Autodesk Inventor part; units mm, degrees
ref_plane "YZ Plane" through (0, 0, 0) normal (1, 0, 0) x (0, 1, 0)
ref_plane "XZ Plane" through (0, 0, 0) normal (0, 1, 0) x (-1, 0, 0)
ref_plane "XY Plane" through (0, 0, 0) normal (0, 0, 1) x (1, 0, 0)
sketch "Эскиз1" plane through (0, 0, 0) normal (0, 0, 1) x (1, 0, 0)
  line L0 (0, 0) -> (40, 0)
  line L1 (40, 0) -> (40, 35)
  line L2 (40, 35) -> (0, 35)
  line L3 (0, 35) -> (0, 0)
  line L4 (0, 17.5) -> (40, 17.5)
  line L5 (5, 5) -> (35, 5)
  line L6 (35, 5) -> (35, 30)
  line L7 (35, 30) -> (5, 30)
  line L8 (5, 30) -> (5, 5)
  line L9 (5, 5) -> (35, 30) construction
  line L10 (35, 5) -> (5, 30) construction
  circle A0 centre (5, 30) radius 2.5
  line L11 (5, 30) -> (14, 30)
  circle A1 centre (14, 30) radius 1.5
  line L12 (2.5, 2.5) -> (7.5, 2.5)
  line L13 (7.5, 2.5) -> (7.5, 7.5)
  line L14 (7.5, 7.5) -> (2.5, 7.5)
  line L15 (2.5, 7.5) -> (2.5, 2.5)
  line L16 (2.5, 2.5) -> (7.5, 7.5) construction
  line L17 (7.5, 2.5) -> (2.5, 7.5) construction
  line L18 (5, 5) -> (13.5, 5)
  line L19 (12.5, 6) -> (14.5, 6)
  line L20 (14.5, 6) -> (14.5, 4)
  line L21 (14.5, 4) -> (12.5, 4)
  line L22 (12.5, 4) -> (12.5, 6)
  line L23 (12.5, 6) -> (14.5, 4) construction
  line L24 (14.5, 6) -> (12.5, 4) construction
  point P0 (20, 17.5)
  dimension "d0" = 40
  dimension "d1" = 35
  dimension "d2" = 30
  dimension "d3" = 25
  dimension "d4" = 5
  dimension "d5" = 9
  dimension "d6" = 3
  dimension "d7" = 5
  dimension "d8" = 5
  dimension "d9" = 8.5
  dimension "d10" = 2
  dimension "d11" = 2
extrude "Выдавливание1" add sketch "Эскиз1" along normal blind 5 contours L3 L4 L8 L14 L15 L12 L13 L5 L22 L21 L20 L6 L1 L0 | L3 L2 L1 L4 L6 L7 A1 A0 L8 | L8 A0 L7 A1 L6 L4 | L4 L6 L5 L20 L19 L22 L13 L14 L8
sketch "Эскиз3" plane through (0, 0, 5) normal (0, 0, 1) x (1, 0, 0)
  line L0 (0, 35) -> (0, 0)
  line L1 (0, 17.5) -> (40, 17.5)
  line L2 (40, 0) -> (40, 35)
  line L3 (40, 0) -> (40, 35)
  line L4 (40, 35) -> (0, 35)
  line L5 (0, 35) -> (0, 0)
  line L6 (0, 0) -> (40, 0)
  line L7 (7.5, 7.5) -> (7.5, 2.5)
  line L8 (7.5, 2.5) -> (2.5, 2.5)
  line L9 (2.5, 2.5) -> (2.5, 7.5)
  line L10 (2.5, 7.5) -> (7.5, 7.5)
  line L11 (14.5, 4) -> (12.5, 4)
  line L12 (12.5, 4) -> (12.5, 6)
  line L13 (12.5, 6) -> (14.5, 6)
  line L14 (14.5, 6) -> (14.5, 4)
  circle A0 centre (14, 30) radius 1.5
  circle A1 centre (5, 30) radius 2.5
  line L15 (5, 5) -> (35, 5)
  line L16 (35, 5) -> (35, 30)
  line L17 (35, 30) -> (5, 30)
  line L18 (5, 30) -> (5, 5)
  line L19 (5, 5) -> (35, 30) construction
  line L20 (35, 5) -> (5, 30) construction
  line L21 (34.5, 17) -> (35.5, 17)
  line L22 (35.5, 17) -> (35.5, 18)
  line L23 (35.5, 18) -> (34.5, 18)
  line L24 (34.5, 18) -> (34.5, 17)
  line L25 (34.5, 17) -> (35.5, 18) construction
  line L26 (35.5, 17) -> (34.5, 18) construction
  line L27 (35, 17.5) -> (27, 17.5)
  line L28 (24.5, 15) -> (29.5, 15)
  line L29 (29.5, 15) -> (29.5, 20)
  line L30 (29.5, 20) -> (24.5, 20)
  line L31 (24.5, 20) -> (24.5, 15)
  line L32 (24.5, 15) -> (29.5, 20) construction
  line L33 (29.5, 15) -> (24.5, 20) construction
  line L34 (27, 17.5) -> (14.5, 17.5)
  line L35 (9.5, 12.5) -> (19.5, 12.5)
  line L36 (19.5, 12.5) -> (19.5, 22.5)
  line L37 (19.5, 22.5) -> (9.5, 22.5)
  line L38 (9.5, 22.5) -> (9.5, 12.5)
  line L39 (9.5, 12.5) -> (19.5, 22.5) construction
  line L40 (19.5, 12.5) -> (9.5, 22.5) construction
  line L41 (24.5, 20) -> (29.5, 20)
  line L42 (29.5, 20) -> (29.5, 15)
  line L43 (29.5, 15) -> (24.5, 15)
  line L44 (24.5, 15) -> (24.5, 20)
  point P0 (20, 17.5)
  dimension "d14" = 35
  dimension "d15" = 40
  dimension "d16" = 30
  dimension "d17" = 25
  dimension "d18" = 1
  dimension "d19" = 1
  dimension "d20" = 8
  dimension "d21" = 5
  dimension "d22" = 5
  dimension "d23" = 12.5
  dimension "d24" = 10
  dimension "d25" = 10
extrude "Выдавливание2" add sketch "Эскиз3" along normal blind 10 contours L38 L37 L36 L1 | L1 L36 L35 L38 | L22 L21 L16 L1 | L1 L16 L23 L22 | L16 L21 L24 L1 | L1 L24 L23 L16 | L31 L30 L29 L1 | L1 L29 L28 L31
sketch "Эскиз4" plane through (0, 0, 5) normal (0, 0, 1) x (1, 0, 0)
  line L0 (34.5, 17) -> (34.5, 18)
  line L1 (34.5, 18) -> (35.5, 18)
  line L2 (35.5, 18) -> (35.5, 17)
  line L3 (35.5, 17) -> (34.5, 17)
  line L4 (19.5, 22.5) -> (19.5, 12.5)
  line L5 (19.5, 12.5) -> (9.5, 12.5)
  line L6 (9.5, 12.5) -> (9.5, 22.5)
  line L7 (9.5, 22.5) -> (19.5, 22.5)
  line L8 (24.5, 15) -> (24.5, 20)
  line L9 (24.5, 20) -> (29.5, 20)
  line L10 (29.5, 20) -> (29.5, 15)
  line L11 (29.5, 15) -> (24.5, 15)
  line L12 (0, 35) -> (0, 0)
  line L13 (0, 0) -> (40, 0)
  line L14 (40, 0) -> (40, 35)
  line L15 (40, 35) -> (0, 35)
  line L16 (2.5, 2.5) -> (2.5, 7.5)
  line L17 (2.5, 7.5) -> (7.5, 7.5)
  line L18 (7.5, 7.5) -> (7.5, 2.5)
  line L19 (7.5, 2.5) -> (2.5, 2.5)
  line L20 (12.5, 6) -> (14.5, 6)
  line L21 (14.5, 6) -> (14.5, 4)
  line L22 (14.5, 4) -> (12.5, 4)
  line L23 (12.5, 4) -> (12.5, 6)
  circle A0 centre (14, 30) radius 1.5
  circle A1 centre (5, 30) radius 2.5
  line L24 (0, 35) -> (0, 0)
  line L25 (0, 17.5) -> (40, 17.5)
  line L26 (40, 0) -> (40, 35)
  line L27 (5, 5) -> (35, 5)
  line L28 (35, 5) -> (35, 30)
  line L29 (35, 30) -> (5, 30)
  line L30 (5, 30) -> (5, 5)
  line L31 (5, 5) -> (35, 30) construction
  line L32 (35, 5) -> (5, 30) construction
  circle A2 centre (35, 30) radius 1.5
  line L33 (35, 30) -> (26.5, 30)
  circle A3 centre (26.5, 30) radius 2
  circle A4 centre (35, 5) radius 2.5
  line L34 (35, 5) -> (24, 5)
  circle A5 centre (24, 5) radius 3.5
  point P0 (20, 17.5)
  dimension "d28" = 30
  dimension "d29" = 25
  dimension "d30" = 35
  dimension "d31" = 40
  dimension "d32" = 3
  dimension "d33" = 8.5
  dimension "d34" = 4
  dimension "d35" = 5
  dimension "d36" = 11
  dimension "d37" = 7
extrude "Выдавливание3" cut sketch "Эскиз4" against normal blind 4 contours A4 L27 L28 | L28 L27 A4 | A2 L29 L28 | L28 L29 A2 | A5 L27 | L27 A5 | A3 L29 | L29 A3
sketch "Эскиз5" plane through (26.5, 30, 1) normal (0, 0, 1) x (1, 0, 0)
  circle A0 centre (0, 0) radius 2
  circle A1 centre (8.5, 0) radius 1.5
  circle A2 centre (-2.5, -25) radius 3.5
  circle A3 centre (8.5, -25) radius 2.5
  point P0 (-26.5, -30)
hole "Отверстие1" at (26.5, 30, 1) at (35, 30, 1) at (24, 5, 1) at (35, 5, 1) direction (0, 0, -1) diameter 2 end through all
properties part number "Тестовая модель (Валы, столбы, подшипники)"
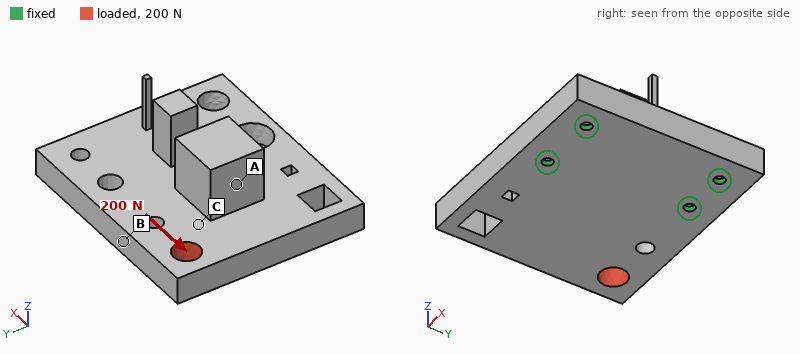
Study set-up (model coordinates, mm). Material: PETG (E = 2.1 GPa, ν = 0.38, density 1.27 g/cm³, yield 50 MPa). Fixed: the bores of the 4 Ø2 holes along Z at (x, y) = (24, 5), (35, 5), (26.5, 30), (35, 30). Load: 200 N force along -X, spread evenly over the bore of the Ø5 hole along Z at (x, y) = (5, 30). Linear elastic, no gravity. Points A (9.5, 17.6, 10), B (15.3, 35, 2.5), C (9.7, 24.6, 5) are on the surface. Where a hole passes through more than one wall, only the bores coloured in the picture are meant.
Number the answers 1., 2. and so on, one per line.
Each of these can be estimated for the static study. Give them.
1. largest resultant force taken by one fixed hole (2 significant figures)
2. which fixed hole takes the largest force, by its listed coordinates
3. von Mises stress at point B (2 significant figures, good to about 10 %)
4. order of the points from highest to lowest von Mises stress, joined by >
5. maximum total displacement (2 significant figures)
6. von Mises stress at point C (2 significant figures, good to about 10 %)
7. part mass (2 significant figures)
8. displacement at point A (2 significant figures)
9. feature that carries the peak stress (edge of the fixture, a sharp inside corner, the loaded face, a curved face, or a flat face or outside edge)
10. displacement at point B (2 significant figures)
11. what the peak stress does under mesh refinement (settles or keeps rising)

1. 120 N
2. (26.5, 30)
3. 4.5 MPa
4. B > C > A
5. 0.14 mm
6. 2.6 MPa
7. 9.7 g
8. 0.071 mm
9. edge of the fixture
10. 0.080 mm
11. keeps rising
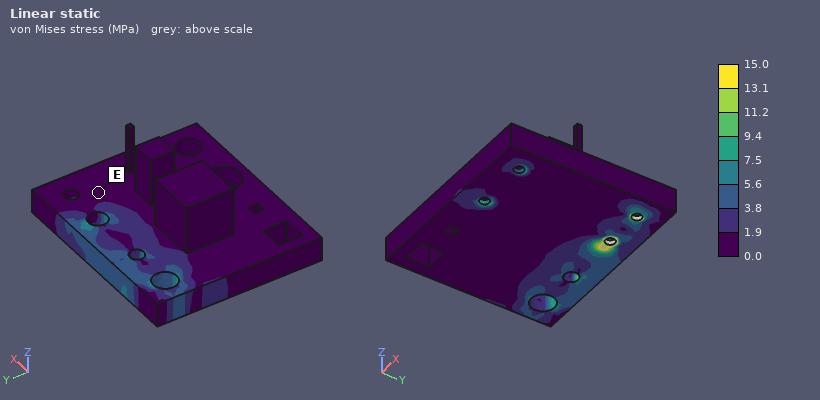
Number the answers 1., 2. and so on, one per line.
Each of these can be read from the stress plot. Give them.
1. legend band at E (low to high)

1. 0.0 to 1.9 MPa
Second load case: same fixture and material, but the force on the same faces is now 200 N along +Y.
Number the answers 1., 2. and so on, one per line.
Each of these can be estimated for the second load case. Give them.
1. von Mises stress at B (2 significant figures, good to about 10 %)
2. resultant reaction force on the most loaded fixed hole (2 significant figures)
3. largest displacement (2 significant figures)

1. 3.4 MPa
2. 140 N
3. 0.15 mm
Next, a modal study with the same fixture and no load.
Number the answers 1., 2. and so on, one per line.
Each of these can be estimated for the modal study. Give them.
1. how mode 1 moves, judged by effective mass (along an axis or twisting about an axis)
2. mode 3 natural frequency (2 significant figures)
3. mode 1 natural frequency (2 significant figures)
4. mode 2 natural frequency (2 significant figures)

1. along Z
2. 2000 Hz
3. 910 Hz
4. 2000 Hz
